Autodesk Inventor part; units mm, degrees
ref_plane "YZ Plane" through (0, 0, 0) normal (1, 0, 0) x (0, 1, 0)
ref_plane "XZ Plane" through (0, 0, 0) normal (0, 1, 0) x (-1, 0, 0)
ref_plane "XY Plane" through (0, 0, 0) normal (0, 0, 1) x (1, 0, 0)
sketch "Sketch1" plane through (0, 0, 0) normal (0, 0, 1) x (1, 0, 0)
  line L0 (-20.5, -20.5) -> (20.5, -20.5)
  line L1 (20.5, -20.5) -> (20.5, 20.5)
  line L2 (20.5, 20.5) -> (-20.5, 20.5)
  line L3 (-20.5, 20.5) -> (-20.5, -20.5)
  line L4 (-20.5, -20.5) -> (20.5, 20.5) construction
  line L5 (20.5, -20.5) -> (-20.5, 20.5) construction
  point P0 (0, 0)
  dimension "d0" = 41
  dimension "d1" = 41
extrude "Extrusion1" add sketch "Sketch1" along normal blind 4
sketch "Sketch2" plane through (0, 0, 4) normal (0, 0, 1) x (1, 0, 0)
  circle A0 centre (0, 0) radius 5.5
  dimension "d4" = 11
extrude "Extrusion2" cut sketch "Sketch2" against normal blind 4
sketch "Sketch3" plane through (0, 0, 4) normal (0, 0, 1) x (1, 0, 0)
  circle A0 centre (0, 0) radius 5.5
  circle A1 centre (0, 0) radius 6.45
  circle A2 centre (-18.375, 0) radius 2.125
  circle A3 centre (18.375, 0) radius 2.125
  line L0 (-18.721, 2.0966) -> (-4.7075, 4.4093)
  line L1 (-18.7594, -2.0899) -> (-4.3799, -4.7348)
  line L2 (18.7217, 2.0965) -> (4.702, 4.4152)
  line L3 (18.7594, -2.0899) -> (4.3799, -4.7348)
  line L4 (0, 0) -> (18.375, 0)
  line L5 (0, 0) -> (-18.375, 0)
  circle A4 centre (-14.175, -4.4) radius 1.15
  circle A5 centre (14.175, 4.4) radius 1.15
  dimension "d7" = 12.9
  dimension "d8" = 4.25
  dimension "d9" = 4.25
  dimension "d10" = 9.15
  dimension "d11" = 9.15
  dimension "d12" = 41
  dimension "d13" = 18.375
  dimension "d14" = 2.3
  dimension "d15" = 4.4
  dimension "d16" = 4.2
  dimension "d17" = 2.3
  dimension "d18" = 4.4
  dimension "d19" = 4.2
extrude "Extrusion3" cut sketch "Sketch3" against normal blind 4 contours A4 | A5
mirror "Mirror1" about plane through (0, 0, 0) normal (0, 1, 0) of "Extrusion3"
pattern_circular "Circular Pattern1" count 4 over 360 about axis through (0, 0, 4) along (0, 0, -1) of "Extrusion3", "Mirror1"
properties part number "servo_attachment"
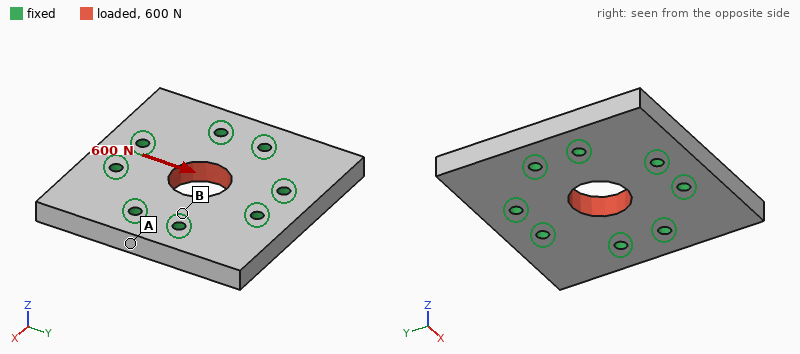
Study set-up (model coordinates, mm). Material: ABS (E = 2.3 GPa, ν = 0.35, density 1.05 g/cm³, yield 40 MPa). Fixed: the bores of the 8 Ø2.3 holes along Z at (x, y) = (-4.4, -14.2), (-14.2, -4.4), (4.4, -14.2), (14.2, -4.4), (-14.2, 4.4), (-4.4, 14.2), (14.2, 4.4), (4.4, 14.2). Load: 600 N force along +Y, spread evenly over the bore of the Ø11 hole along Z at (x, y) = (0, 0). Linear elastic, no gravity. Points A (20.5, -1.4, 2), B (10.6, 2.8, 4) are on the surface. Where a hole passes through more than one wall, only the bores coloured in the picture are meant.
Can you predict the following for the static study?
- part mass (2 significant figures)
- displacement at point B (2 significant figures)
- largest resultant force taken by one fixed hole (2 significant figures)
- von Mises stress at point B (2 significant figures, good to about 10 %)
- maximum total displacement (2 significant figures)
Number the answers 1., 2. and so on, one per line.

1. 6.5 g
2. 4.4 µm
3. 110 N
4. 2.1 MPa
5. 19 µm
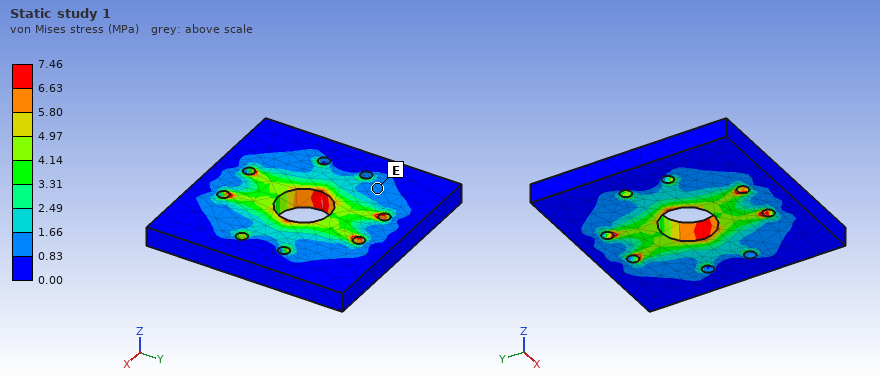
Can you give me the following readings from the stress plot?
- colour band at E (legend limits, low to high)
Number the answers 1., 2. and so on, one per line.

1. 0.83 to 1.66 MPa
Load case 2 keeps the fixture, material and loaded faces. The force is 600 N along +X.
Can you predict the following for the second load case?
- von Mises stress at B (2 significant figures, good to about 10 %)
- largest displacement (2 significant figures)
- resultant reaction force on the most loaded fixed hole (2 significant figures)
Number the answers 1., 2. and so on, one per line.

1. 4.3 MPa
2. 19 µm
3. 110 N
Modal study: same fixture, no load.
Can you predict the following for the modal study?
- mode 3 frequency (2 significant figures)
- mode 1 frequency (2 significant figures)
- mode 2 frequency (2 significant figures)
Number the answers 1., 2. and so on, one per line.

1. 6000 Hz
2. 5900 Hz
3. 6000 Hz
